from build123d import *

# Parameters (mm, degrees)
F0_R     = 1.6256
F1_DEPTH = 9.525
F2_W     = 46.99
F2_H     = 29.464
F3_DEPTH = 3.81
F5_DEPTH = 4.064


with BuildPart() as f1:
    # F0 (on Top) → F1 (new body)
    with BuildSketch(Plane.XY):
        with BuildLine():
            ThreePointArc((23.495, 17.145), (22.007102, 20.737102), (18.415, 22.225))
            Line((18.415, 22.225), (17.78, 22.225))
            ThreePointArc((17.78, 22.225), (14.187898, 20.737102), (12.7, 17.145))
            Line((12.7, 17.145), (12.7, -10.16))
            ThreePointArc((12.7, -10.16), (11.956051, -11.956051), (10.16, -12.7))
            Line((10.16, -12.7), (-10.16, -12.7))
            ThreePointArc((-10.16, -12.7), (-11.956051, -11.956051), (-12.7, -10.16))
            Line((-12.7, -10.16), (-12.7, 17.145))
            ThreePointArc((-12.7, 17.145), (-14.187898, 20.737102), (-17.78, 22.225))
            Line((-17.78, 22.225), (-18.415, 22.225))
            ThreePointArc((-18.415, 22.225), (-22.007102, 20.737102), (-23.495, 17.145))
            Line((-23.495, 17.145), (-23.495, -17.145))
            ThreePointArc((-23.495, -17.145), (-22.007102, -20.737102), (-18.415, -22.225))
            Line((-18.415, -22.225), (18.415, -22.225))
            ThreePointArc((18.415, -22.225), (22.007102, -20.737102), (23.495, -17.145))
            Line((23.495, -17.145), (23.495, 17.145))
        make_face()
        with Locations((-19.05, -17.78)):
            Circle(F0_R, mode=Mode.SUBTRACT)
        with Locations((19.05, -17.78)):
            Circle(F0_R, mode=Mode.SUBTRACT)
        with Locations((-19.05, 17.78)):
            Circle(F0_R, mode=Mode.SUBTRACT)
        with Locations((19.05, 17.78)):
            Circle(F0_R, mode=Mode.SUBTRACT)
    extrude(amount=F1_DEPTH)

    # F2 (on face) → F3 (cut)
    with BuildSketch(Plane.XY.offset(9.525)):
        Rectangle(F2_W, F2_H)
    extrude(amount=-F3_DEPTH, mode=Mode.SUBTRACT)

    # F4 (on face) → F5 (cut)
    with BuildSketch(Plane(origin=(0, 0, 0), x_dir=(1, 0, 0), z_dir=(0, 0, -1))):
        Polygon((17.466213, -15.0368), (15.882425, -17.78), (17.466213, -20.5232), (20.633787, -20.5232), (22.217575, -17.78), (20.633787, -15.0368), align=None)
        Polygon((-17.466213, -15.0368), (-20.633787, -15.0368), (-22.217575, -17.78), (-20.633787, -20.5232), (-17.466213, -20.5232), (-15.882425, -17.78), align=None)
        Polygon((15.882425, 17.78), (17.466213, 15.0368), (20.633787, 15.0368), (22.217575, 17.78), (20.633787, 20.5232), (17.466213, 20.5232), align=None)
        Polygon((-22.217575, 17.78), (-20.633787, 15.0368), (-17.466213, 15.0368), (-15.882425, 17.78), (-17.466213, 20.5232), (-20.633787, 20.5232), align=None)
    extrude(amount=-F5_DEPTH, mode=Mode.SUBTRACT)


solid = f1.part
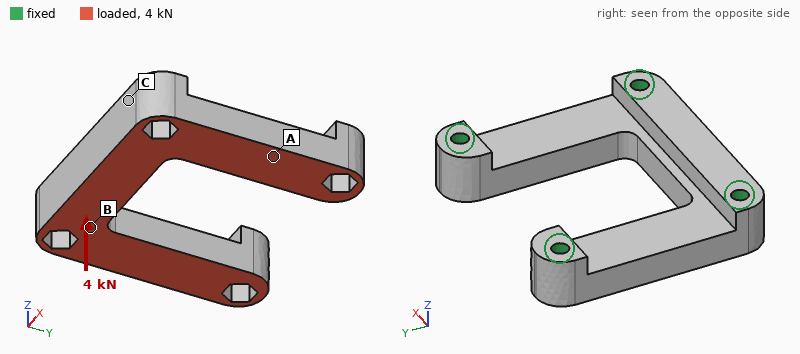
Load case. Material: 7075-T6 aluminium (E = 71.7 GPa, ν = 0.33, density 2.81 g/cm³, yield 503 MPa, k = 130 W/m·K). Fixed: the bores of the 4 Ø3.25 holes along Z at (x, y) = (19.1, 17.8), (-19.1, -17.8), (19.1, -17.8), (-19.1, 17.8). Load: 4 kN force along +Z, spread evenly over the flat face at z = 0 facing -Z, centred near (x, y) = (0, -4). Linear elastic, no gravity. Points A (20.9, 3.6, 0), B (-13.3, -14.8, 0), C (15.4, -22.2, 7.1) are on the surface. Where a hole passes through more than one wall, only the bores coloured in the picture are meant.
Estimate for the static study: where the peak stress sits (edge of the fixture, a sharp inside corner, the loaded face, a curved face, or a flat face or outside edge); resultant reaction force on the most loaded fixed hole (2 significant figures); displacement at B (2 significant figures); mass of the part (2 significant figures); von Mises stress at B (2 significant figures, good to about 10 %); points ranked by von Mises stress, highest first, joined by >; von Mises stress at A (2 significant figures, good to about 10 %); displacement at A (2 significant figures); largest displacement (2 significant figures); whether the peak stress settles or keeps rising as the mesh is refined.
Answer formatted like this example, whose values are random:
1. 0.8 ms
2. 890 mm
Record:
1. edge of the fixture
2. 1.4 kN
3. 9.9 µm
4. 22 g
5. 21 MPa
6. A > B > C
7. 42 MPa
8. 18 µm
9. 24 µm
10. keeps rising
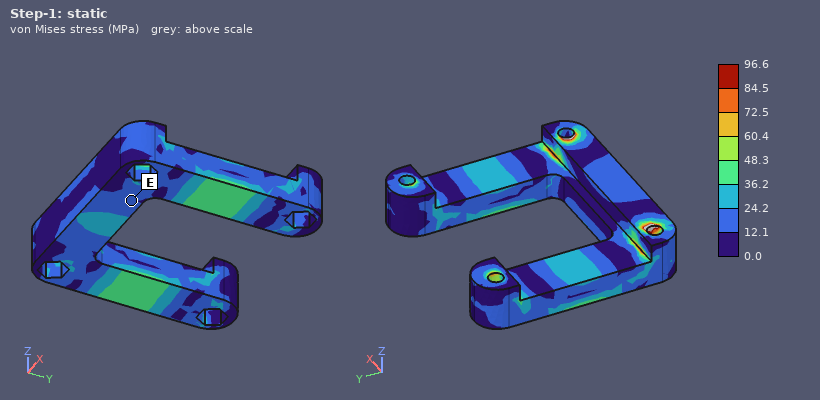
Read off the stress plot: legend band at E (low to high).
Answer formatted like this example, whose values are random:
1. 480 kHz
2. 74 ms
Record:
1. 12.1 to 24.2 MPa
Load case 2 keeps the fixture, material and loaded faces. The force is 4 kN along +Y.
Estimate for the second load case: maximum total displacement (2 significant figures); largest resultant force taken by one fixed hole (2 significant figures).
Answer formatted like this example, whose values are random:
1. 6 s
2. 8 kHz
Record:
1. 20 µm
2. 1.0 kN
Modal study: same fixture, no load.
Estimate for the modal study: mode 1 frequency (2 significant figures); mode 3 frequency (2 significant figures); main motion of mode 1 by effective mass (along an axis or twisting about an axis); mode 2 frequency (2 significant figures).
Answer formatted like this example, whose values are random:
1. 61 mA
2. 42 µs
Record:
1. 18 kHz
2. 20 kHz
3. along Z
4. 19 kHz
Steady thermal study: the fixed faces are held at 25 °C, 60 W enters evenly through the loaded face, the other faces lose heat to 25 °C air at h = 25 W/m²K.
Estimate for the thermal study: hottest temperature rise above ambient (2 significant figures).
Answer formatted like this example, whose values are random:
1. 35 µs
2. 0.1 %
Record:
1. 17 K
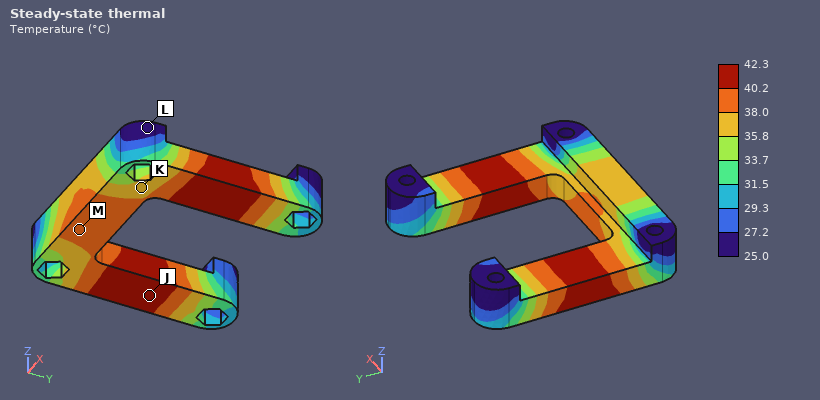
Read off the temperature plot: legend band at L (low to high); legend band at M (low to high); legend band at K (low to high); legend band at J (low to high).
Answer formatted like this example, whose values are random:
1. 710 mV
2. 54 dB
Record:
1. 25.0 to 27.2 °C
2. 38.0 to 40.2 °C
3. 35.8 to 38.0 °C
4. 40.2 to 42.3 °C
